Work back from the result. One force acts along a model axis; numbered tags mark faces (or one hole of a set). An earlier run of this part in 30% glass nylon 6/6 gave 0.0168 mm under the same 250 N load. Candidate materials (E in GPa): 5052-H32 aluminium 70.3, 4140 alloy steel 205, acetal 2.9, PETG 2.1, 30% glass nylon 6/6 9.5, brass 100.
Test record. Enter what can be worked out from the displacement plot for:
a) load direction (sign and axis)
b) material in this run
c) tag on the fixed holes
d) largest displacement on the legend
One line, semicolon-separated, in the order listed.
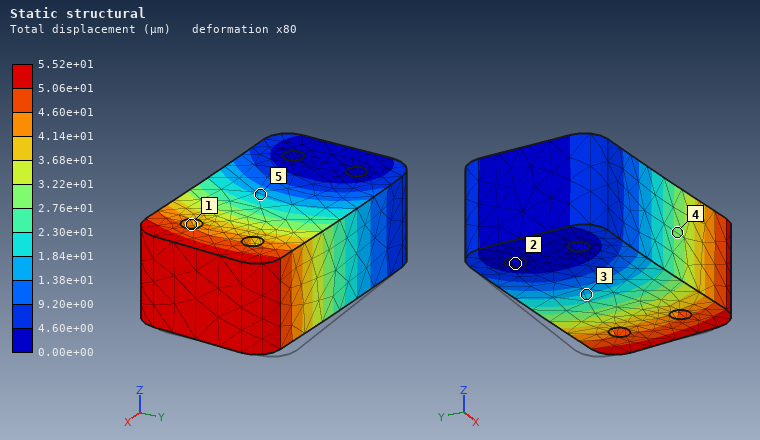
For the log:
-Y; acetal; 2; 5.52e+01 µm
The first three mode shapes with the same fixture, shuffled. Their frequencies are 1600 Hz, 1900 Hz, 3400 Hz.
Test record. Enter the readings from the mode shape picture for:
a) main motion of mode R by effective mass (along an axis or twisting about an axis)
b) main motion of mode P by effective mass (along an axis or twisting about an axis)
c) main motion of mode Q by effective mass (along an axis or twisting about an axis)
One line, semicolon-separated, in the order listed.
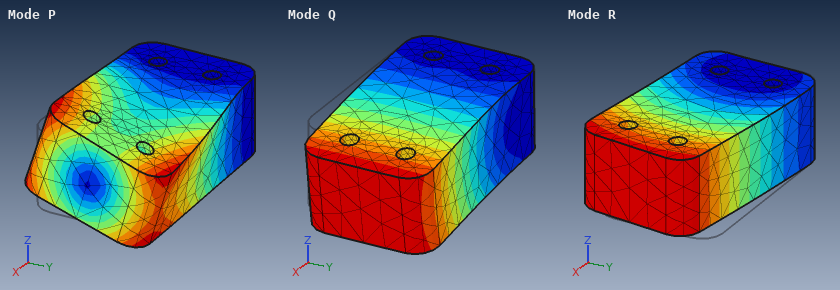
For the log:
along Y; twisting about X; along Z
